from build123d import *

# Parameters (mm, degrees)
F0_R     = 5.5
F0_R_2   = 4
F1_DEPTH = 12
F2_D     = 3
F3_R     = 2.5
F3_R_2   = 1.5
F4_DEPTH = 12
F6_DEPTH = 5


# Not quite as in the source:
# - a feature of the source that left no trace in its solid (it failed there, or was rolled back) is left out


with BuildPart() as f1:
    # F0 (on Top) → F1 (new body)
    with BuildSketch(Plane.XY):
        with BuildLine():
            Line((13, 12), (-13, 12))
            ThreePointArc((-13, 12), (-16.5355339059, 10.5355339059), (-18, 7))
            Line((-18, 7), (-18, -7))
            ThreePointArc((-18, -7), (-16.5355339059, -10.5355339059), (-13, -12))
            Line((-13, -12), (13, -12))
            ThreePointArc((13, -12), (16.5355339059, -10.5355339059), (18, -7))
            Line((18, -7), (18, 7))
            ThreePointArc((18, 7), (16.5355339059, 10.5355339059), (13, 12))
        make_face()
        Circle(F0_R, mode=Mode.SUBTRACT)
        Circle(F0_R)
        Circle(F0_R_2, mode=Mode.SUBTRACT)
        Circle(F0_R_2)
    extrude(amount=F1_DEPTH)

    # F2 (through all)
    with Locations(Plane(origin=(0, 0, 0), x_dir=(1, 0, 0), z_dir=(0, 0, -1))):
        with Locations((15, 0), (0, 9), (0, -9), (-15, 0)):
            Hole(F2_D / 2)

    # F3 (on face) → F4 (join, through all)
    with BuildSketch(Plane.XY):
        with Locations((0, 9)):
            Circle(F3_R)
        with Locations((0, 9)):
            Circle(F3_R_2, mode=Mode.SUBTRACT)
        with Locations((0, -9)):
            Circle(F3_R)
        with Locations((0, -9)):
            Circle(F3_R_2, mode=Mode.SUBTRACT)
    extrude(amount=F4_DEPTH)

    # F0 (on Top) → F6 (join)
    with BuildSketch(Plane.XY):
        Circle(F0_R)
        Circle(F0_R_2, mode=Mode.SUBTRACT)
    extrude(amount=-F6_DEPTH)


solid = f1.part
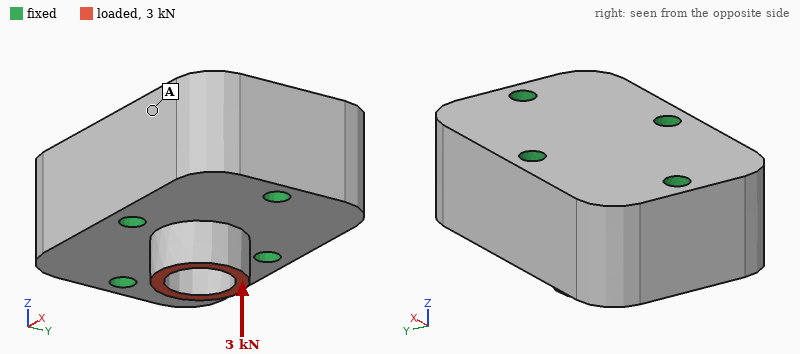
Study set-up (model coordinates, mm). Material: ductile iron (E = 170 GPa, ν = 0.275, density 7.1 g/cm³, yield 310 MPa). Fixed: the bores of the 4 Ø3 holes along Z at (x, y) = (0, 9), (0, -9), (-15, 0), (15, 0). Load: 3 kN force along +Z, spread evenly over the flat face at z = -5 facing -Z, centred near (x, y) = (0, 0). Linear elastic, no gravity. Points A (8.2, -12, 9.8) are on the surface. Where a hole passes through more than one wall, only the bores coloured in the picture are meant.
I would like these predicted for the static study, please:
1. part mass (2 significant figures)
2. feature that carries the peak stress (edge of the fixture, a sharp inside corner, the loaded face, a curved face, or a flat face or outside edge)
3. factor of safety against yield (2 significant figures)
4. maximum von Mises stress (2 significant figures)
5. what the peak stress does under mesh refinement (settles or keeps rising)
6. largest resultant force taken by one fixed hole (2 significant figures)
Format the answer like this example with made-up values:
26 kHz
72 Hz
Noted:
71 g
a curved face
4.0
78 MPa
settles
1.1 kN
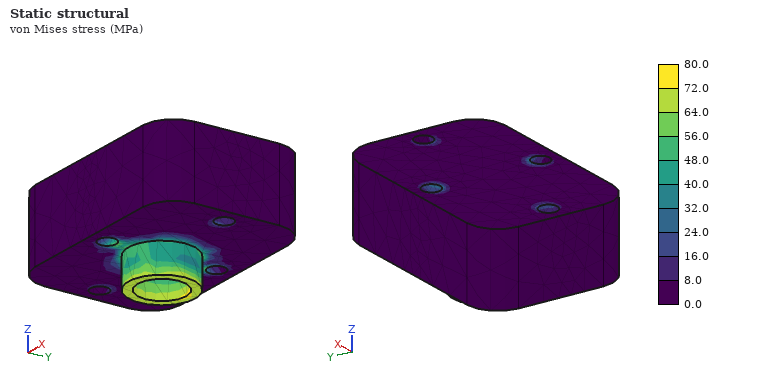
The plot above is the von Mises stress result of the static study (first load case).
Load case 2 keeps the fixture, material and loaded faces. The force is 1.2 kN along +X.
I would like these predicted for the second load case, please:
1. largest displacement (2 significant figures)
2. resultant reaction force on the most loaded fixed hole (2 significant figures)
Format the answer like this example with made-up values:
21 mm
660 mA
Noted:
9.4 µm
430 N
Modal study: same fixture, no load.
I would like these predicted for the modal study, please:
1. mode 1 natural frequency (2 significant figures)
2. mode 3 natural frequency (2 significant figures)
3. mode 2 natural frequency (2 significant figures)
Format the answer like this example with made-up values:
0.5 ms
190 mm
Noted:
54 kHz
55 kHz
55 kHz
